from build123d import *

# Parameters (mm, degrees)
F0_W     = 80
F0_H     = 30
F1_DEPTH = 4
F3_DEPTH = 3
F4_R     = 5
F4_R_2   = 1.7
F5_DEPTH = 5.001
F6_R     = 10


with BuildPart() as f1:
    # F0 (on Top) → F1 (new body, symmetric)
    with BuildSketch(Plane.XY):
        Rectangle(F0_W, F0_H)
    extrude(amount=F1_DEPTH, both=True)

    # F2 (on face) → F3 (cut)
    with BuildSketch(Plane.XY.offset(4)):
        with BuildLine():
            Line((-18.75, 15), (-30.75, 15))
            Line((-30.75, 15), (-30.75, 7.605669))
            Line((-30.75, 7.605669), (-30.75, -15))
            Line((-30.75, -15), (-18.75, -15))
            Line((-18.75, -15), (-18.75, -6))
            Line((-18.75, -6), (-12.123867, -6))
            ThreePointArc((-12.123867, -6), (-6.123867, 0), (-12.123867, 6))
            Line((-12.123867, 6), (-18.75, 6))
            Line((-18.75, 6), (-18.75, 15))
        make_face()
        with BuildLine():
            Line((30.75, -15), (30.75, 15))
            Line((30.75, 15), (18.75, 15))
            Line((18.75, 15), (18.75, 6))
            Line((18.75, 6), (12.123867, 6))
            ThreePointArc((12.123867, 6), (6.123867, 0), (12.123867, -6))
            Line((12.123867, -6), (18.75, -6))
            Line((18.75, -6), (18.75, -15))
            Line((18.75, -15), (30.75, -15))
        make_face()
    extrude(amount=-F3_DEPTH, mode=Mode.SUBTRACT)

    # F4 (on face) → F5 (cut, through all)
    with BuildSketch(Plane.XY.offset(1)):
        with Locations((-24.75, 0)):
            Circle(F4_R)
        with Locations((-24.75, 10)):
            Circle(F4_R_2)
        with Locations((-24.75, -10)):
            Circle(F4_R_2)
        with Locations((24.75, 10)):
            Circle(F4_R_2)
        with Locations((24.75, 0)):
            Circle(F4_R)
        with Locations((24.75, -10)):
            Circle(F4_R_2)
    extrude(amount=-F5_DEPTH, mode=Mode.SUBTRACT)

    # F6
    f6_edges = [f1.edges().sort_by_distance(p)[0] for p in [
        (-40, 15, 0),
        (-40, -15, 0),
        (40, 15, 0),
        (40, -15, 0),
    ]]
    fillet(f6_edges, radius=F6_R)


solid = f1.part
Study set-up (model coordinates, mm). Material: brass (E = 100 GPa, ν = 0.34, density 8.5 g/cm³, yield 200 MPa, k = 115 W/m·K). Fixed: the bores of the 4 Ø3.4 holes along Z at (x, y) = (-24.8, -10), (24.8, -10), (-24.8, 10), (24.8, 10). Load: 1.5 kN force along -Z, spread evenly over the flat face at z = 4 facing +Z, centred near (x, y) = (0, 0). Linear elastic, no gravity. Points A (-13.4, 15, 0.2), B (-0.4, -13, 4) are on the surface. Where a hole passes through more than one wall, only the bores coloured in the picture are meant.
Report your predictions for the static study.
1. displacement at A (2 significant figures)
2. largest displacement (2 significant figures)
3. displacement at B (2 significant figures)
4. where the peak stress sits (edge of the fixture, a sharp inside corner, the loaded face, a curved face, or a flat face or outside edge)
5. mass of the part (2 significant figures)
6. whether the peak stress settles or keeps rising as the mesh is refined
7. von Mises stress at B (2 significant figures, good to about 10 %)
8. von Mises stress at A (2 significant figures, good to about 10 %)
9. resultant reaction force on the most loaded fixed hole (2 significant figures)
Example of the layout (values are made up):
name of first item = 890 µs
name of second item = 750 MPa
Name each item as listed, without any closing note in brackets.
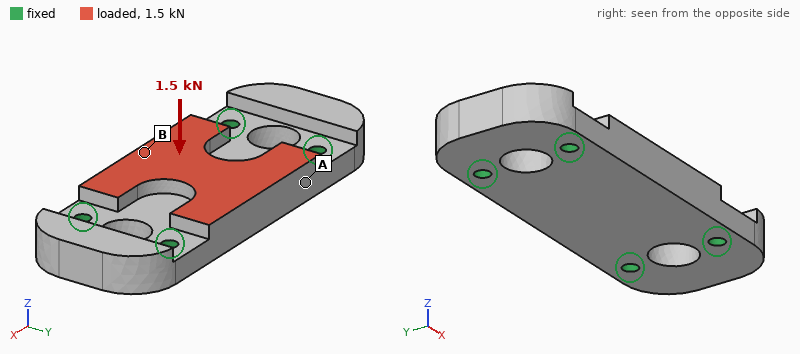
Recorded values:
displacement at A = 8.0 µm
largest displacement = 13 µm
displacement at B = 13 µm
where the peak stress sits = edge of the fixture
mass of the part = 120 g
whether the peak stress settles or keeps rising as the mesh is refined = keeps rising
von Mises stress at B = 25 MPa
von Mises stress at A = 12 MPa
resultant reaction force on the most loaded fixed hole = 470 N
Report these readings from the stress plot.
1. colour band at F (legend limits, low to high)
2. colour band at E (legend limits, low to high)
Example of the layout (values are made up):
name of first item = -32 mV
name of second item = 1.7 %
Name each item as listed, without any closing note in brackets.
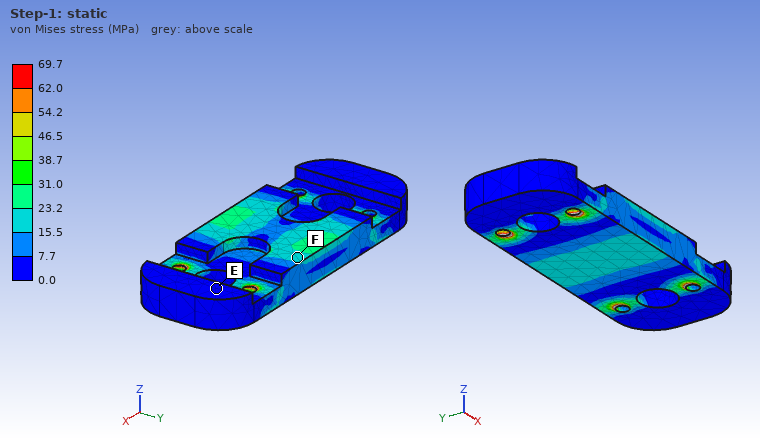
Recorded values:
colour band at F = 15.5 to 23.2 MPa
colour band at E = 0.0 to 7.7 MPa
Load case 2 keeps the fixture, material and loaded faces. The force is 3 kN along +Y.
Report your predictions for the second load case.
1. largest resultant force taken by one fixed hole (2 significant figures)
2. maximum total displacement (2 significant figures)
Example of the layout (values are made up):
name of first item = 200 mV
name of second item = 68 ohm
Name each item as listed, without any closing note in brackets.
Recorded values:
largest resultant force taken by one fixed hole = 1.1 kN
maximum total displacement = 19 µm
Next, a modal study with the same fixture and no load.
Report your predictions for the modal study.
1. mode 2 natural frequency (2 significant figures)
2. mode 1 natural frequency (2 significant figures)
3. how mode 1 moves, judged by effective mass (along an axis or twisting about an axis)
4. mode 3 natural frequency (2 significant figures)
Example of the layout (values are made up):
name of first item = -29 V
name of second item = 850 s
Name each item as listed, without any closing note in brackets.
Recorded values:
mode 2 natural frequency = 8700 Hz
mode 1 natural frequency = 7300 Hz
how mode 1 moves, judged by effective mass = along Z
mode 3 natural frequency = 8800 Hz
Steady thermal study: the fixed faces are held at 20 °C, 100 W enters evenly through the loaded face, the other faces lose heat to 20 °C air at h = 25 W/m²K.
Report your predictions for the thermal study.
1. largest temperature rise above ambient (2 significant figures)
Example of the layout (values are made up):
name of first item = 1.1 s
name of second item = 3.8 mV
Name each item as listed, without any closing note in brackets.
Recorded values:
largest temperature rise above ambient = 49 K
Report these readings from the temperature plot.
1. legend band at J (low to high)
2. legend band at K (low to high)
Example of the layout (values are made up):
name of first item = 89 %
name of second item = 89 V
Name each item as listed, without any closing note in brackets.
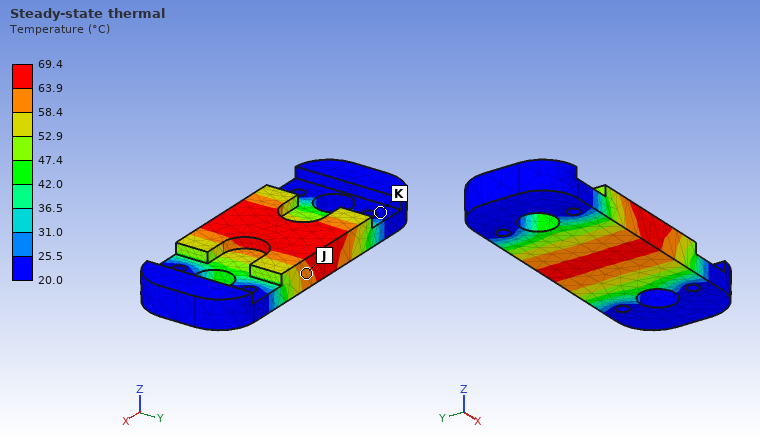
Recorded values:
legend band at J = 58.4 to 63.9 °C
legend band at K = 20.0 to 25.5 °C
